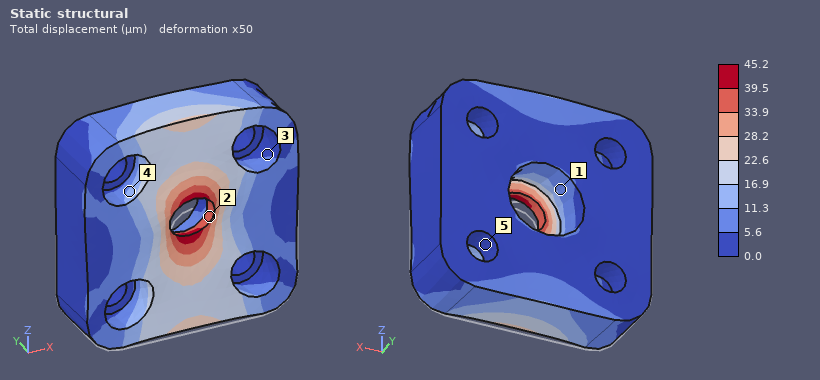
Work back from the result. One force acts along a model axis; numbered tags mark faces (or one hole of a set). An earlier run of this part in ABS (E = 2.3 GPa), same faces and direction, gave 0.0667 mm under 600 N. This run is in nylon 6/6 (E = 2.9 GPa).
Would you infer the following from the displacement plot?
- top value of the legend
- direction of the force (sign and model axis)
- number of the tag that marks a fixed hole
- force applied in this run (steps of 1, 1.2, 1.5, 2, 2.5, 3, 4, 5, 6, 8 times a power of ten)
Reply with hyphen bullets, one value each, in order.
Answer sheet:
- 45.2 µm
- +Z
- 5
- 500 N
